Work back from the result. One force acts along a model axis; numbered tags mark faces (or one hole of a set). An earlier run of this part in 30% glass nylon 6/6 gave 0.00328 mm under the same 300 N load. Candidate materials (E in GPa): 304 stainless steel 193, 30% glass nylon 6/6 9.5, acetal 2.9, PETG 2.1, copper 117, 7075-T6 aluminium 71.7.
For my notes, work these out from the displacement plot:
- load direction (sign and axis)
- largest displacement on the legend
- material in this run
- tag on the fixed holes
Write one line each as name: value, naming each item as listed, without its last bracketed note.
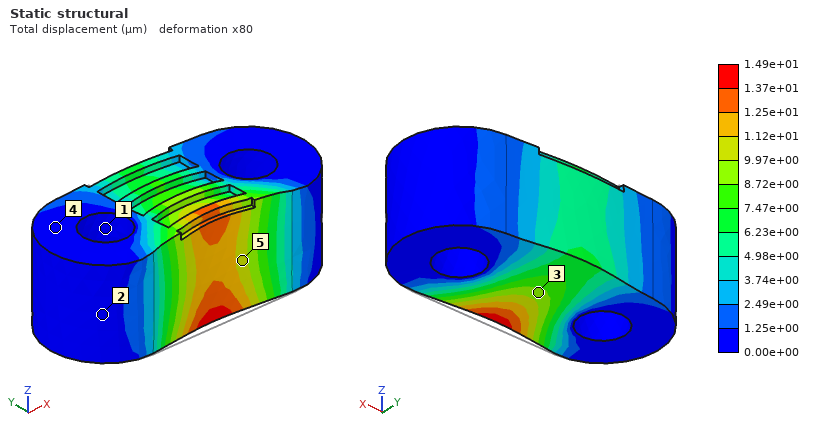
load direction: +Y
largest displacement on the legend: 1.49e+01 µm
material in this run: PETG
tag on the fixed holes: 1
